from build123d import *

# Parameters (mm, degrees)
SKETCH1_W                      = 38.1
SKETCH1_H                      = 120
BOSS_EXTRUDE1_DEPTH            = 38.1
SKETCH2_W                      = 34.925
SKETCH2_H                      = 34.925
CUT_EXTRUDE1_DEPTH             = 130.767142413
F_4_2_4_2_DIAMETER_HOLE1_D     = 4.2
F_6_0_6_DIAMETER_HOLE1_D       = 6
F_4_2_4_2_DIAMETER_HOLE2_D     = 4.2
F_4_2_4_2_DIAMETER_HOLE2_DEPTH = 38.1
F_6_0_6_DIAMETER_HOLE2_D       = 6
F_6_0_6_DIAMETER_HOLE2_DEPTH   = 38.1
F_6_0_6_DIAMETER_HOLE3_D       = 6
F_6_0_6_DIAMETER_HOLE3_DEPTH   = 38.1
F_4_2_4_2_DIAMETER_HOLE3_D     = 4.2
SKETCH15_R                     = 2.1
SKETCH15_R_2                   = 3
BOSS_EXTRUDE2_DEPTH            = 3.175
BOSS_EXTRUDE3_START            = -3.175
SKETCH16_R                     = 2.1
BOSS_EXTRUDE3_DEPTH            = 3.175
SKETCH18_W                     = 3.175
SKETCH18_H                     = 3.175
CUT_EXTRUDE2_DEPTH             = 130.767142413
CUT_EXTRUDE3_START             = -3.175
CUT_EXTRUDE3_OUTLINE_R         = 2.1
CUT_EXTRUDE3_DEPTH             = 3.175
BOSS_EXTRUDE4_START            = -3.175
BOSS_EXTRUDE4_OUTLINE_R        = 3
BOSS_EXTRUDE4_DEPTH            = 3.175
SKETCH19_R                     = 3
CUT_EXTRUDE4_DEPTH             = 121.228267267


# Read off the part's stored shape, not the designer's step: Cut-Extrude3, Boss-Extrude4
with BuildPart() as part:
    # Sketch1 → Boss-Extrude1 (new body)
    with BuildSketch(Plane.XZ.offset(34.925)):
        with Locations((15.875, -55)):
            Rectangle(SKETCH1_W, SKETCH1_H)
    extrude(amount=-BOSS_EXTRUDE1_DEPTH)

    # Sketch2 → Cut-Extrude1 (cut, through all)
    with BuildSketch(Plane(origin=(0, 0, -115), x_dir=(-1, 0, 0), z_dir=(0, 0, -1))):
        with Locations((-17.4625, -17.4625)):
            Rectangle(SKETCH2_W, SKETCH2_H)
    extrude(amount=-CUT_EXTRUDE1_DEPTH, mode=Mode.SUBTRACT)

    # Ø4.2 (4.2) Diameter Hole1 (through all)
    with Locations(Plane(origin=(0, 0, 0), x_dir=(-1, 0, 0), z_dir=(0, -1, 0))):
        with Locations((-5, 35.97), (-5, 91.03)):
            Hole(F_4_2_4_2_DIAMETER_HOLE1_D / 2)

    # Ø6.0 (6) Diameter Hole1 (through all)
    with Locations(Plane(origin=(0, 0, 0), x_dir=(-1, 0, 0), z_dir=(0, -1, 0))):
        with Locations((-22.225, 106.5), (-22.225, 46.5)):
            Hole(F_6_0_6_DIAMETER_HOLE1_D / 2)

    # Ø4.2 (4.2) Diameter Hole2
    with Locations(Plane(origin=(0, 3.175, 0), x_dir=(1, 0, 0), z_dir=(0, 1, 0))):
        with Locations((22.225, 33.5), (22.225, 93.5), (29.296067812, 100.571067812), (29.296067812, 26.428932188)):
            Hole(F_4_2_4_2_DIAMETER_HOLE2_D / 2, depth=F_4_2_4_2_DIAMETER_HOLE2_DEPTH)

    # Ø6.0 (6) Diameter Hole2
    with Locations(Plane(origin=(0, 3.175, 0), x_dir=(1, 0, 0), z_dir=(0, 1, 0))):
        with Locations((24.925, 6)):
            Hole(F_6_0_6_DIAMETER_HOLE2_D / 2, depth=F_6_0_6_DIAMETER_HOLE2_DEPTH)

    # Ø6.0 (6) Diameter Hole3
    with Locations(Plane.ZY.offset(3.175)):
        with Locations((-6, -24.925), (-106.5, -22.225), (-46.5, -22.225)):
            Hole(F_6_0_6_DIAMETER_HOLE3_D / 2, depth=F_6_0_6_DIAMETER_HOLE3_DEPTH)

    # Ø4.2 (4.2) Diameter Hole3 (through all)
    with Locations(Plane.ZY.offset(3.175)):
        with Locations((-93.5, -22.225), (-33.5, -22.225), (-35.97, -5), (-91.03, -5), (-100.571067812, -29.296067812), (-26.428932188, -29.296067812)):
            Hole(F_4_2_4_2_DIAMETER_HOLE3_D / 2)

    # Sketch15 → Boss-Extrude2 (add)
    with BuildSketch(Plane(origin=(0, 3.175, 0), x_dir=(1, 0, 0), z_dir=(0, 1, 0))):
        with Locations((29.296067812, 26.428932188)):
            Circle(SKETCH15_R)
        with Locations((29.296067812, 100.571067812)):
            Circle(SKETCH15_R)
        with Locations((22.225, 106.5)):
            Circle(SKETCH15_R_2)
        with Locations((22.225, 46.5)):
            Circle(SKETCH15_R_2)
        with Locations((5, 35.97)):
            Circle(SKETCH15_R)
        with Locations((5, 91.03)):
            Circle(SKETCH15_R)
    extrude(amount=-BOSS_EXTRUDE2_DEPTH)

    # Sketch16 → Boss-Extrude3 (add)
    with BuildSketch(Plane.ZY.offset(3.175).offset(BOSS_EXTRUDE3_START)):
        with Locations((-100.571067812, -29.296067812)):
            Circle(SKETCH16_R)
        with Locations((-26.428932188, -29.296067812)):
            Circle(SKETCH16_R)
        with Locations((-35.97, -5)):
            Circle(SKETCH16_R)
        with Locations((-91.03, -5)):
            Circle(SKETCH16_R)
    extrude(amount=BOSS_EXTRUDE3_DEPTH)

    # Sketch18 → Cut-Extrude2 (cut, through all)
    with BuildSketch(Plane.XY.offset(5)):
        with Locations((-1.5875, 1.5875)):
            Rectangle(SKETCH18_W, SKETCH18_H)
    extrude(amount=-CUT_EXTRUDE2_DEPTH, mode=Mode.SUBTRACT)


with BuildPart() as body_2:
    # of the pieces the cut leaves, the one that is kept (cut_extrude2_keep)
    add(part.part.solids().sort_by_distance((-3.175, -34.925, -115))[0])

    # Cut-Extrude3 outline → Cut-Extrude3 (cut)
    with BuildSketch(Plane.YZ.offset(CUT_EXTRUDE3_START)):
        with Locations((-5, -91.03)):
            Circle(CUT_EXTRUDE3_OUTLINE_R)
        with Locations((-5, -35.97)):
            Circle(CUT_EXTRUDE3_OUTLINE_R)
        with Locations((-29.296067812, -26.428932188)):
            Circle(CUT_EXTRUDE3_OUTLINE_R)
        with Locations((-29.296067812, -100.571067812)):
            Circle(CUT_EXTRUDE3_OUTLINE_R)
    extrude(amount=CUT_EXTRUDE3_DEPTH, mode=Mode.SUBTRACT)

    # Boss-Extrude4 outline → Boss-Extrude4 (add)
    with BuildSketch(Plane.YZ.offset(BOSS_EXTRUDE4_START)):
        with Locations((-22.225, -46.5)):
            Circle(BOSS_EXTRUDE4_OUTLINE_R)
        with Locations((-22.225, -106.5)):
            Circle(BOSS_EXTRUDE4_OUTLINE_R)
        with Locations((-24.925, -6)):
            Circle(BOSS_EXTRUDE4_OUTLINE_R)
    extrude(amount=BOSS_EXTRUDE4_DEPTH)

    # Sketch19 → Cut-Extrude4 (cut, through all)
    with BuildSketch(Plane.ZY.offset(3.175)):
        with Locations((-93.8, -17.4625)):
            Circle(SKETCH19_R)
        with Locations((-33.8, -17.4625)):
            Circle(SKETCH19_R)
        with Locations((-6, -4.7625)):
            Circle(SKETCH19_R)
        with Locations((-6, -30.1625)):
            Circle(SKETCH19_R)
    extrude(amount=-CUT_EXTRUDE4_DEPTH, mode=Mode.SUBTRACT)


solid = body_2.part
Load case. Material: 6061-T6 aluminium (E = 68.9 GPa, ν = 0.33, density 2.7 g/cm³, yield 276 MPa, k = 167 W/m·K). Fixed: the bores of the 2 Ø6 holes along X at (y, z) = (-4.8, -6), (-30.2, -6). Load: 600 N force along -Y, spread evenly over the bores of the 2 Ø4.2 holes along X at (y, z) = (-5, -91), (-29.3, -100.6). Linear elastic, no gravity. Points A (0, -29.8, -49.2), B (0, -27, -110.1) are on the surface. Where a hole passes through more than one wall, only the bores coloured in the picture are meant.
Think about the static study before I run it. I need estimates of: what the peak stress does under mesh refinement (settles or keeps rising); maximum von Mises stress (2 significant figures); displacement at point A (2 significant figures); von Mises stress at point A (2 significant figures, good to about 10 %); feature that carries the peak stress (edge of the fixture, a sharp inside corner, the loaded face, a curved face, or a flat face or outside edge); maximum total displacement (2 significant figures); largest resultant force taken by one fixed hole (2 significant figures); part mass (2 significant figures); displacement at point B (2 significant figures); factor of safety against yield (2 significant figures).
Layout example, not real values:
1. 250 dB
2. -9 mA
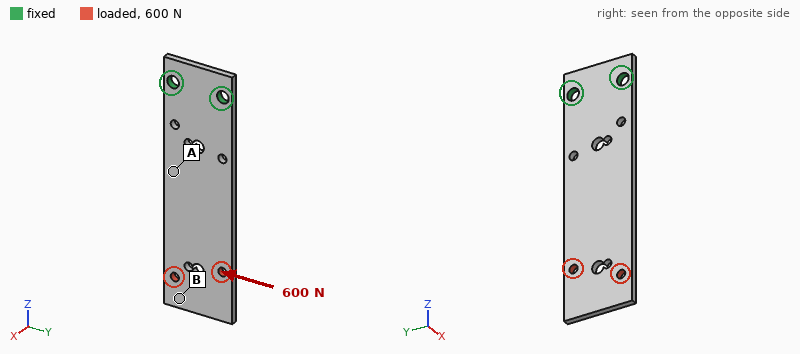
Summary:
1. settles
2. 170 MPa
3. 0.073 mm
4. 33 MPa
5. a curved face
6. 0.29 mm
7. 2.0 kN
8. 34 g
9. 0.27 mm
10. 1.6
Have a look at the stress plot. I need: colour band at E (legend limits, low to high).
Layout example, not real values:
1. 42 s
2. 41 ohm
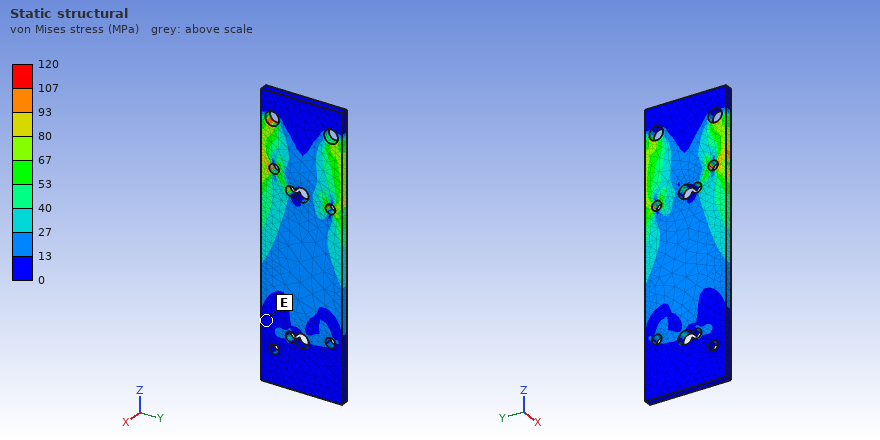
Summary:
1. 0 to 13 MPa
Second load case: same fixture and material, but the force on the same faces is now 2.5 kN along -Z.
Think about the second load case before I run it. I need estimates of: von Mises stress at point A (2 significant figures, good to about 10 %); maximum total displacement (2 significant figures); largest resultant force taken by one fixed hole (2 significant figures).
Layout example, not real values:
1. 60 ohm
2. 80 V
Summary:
1. 23 MPa
2. 39 µm
3. 1.3 kN
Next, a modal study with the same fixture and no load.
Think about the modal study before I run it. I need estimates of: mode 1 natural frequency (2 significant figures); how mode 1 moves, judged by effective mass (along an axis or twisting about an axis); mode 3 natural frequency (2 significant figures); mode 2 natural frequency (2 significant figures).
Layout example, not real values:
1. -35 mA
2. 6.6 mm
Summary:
1. 220 Hz
2. along X
3. 1400 Hz
4. 1400 Hz
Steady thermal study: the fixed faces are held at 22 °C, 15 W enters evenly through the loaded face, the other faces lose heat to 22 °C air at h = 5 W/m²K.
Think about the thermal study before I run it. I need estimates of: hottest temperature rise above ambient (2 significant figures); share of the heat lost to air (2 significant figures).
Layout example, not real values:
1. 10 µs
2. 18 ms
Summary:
1. 77 K
2. 12 %
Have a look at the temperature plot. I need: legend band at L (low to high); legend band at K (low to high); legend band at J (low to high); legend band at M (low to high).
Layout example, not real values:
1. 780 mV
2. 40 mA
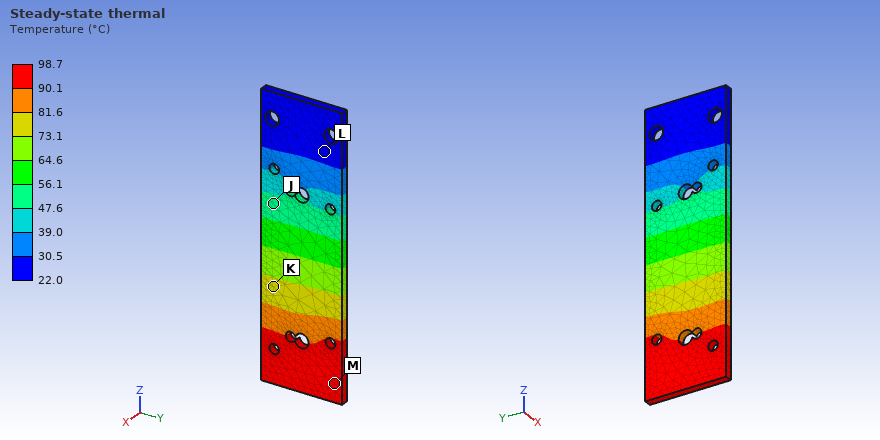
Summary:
1. 22.0 to 30.5 °C
2. 73.1 to 81.6 °C
3. 47.6 to 56.1 °C
4. 90.1 to 98.7 °C
